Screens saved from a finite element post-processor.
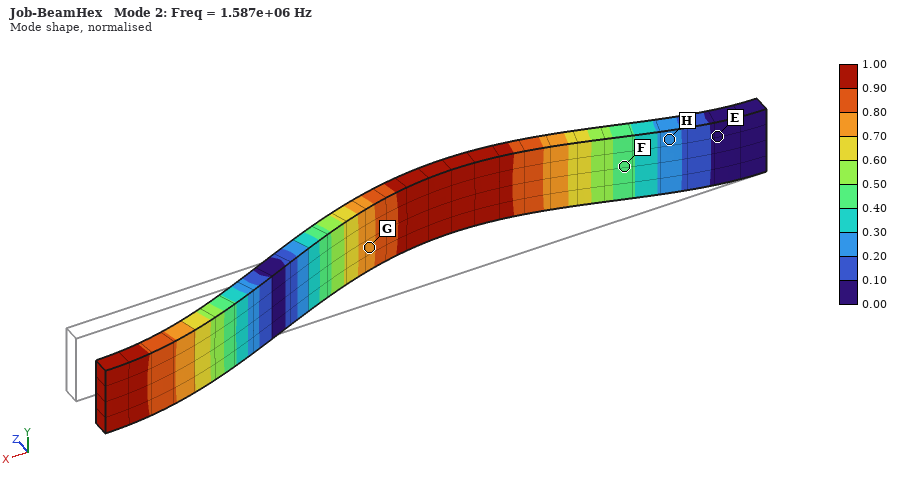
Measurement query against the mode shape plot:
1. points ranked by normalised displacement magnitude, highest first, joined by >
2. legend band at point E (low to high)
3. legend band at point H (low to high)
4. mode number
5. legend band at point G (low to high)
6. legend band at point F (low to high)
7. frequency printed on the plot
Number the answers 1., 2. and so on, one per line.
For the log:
1. G > F > H > E
2. 0.00 to 0.10
3. 0.20 to 0.30
4. 2
5. 0.70 to 0.80
6. 0.40 to 0.50
7. 1.587e+06 Hz
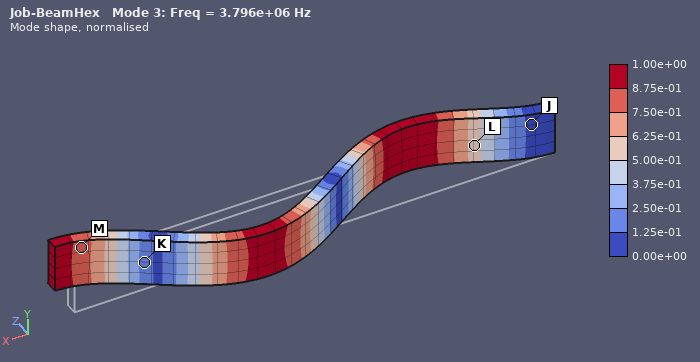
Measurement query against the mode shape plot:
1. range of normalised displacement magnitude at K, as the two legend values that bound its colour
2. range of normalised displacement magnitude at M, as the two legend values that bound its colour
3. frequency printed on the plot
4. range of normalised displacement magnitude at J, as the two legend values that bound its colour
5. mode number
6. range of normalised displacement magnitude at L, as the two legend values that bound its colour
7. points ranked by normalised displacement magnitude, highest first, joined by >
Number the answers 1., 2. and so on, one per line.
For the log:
1. 1.25e-01 to 2.50e-01
2. 7.50e-01 to 8.75e-01
3. 3.796e+06 Hz
4. 0.00e+00 to 1.25e-01
5. 3
6. 5.00e-01 to 6.25e-01
7. M > L > K > J
